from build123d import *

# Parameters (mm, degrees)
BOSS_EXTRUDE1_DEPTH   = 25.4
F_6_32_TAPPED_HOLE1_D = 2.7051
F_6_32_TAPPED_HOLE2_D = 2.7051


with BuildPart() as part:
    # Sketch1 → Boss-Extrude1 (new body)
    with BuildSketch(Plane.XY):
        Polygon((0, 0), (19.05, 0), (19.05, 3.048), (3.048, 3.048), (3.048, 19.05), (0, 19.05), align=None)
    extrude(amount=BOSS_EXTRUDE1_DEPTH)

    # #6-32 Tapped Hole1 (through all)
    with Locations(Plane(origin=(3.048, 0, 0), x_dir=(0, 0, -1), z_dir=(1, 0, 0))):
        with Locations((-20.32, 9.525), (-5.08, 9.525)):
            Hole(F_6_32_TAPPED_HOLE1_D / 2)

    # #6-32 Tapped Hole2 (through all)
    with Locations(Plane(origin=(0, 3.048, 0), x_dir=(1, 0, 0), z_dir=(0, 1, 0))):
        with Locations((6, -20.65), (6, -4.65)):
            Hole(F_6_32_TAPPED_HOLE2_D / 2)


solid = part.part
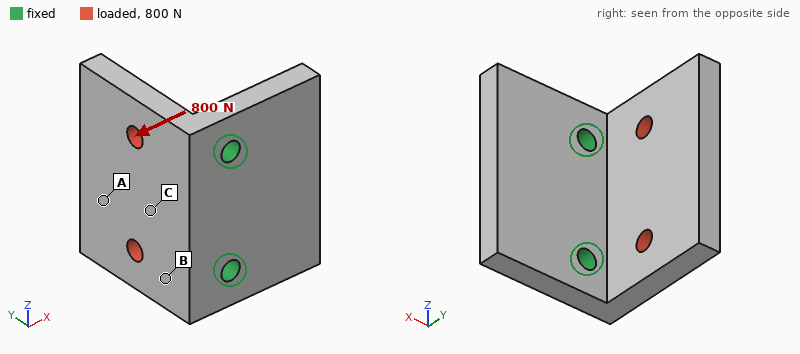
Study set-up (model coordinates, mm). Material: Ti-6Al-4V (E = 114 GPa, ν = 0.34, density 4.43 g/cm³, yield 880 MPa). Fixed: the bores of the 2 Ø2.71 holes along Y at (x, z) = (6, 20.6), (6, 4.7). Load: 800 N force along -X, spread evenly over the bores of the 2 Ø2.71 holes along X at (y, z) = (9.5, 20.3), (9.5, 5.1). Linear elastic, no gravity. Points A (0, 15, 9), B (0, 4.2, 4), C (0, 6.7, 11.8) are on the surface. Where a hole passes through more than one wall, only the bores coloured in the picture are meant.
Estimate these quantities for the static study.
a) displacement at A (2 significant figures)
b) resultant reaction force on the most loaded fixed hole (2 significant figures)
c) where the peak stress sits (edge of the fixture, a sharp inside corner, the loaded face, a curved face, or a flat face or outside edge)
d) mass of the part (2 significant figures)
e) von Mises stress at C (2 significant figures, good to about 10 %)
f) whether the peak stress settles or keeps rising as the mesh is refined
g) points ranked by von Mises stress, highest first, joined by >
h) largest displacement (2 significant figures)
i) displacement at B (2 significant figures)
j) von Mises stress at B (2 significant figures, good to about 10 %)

0.084 mm
400 N
edge of the fixture
12 g
53 MPa
keeps rising
B > C > A
0.11 mm
0.021 mm
100 MPa
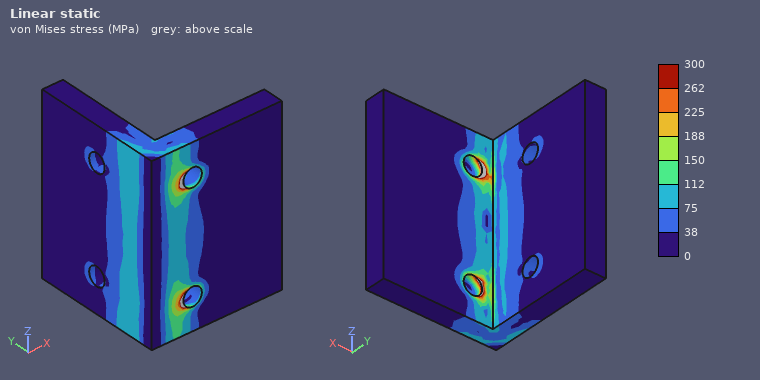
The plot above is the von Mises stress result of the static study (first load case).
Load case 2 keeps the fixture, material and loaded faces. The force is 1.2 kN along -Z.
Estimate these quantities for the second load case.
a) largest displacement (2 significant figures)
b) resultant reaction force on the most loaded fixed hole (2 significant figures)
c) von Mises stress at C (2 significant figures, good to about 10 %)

21 µm
850 N
19 MPa
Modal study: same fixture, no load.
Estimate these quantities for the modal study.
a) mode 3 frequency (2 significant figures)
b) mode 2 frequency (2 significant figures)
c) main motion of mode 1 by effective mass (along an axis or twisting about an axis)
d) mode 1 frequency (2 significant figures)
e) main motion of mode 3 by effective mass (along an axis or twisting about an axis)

14 kHz
12 kHz
along X
6000 Hz
along Y
